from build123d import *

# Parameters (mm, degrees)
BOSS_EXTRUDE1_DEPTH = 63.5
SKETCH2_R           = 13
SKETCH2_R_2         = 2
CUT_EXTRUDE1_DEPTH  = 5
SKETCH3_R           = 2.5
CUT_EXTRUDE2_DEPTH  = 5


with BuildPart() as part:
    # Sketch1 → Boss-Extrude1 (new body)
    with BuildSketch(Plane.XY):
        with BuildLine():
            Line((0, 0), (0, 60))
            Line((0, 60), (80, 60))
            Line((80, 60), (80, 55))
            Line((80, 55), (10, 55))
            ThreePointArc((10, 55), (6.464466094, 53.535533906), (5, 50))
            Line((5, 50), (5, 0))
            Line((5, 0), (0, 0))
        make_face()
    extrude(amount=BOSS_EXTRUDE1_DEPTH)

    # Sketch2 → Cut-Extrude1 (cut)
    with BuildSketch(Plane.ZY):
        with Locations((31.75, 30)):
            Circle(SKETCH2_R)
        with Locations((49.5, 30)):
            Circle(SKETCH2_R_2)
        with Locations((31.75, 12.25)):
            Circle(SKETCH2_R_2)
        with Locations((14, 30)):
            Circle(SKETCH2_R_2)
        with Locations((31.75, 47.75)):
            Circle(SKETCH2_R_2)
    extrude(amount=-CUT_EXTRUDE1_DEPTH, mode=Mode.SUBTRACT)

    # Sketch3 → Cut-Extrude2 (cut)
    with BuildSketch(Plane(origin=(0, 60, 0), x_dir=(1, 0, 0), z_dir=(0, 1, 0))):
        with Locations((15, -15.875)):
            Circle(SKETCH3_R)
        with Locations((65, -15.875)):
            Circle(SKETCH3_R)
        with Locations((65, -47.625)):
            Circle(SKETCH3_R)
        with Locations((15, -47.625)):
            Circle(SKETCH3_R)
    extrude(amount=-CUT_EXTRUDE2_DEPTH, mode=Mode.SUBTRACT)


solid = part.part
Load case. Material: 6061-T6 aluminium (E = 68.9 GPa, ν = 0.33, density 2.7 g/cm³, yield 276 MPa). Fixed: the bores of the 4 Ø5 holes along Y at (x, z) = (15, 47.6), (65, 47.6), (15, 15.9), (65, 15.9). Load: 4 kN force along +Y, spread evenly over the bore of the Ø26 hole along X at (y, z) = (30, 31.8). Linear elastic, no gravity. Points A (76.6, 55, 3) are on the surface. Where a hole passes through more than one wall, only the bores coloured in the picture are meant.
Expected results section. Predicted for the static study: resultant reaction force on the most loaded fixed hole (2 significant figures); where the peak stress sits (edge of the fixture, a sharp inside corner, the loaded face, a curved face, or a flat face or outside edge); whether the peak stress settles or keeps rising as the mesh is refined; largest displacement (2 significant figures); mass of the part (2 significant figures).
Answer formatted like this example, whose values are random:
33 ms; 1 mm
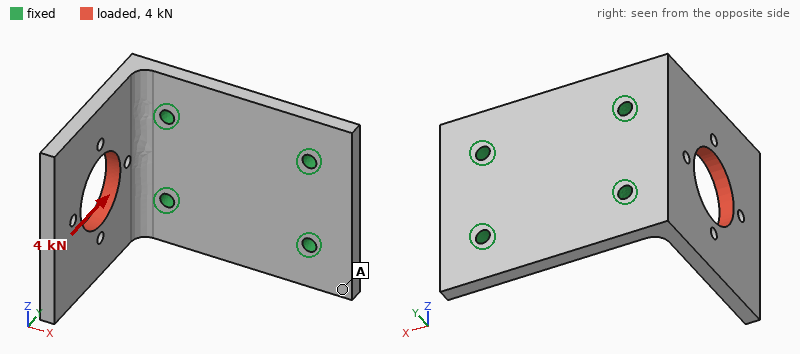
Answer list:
2.1 kN; edge of the fixture; keeps rising; 0.42 mm; 110 g
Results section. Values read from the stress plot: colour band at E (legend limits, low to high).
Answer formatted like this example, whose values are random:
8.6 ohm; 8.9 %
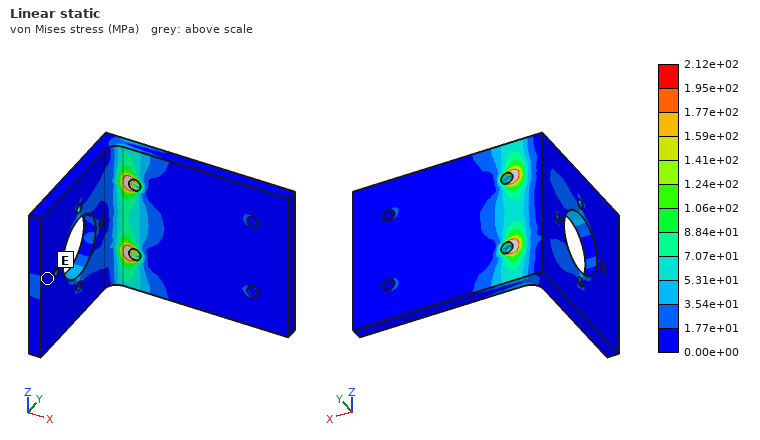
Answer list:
0.00e+00 to 1.77e+01 MPa
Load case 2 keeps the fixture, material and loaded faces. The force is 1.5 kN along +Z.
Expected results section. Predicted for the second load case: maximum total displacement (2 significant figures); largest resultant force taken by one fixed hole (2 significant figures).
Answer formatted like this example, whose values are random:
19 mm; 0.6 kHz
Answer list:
0.13 mm; 1.4 kN
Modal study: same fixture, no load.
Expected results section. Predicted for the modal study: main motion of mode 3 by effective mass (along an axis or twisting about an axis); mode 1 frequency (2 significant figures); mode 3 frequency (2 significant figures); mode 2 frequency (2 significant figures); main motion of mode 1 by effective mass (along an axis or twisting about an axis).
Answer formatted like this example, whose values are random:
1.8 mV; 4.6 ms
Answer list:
along Z; 980 Hz; 3400 Hz; 2200 Hz; along X
